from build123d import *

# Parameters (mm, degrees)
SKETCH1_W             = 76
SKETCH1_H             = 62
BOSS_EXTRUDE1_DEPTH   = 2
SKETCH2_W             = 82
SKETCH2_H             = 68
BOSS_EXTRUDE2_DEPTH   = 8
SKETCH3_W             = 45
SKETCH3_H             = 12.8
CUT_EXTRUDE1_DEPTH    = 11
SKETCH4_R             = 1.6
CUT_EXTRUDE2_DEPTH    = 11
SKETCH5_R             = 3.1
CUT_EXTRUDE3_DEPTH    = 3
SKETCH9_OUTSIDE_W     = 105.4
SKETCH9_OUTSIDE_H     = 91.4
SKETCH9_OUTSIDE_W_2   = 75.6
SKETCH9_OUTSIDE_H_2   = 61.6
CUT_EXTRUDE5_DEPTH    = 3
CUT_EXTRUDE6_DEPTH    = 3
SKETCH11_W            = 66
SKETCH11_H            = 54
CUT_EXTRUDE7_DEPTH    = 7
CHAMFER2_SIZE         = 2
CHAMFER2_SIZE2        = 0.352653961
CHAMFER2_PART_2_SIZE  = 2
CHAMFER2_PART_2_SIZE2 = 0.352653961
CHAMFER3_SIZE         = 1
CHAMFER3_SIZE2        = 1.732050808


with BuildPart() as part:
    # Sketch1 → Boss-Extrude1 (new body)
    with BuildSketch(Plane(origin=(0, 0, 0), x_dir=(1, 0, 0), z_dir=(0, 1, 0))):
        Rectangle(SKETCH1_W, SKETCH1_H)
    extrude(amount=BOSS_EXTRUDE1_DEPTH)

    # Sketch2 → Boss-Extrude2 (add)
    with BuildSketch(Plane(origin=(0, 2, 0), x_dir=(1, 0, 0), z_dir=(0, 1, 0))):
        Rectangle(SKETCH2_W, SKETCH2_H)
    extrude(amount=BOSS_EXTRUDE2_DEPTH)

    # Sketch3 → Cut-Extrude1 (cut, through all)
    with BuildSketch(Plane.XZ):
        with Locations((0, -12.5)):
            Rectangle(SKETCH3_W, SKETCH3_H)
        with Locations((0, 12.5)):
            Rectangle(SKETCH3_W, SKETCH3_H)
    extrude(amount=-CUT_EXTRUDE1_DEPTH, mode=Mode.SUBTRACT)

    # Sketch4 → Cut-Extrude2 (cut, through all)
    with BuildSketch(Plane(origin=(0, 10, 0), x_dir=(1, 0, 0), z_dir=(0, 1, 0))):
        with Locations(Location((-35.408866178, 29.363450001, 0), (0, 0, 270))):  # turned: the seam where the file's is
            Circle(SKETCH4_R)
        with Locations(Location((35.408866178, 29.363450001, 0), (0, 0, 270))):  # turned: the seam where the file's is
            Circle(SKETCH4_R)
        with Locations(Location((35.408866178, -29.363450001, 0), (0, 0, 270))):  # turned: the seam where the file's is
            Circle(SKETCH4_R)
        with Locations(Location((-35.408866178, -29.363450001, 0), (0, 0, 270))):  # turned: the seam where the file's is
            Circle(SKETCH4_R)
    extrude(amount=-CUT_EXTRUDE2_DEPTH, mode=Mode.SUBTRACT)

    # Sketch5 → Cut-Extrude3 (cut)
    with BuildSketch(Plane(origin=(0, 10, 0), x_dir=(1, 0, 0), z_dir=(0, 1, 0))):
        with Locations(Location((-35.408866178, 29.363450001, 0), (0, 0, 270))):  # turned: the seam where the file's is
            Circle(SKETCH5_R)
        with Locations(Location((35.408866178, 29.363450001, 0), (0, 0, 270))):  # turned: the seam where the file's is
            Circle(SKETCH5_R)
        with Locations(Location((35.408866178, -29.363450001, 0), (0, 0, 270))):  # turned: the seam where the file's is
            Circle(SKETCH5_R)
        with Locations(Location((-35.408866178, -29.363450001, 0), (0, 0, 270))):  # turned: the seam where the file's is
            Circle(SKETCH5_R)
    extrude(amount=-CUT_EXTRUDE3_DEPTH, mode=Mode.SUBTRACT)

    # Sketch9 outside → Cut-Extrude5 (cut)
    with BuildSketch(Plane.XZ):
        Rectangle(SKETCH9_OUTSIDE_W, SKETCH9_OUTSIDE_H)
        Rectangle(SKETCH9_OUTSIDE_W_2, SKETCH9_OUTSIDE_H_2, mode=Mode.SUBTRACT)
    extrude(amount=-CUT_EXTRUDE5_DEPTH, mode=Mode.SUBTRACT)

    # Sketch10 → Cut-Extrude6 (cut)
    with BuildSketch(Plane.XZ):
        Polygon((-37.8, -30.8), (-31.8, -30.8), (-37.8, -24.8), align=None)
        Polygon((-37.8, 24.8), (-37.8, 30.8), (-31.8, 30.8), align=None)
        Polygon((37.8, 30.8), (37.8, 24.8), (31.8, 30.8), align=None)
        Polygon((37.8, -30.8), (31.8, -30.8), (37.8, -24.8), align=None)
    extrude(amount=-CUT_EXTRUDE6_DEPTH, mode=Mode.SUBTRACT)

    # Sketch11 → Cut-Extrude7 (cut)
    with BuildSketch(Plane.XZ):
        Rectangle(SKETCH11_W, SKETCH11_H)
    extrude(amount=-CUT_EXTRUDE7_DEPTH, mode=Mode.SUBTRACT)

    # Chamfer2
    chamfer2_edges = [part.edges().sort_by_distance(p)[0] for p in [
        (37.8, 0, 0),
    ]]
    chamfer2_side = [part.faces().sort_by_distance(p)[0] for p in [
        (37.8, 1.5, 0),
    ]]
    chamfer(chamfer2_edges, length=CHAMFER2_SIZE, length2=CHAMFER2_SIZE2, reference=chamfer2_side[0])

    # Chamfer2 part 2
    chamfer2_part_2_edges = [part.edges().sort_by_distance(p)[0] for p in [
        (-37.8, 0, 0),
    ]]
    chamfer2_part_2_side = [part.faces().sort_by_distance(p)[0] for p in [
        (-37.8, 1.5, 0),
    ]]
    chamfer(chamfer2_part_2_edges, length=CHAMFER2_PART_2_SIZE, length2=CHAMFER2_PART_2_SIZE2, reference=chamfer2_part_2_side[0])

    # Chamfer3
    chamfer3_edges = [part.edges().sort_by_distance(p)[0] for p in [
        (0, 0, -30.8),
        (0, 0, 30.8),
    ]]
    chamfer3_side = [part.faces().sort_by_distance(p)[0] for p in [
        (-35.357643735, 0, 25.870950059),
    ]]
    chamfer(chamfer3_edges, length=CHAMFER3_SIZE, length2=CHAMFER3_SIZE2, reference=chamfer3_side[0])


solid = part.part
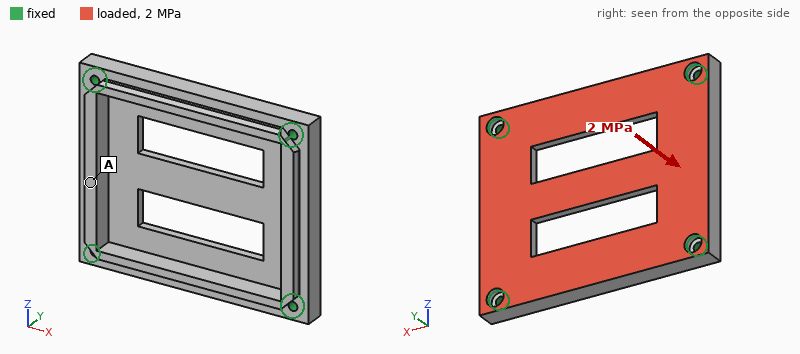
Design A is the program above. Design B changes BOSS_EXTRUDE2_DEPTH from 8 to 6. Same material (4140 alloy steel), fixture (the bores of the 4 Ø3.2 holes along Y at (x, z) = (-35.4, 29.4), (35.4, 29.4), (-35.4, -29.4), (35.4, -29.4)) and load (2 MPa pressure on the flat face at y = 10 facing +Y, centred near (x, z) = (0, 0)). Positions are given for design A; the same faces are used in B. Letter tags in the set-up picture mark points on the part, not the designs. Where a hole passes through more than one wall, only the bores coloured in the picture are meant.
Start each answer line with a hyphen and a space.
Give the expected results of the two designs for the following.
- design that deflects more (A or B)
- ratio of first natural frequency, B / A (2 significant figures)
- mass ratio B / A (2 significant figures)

- B
- 0.40
- 0.64
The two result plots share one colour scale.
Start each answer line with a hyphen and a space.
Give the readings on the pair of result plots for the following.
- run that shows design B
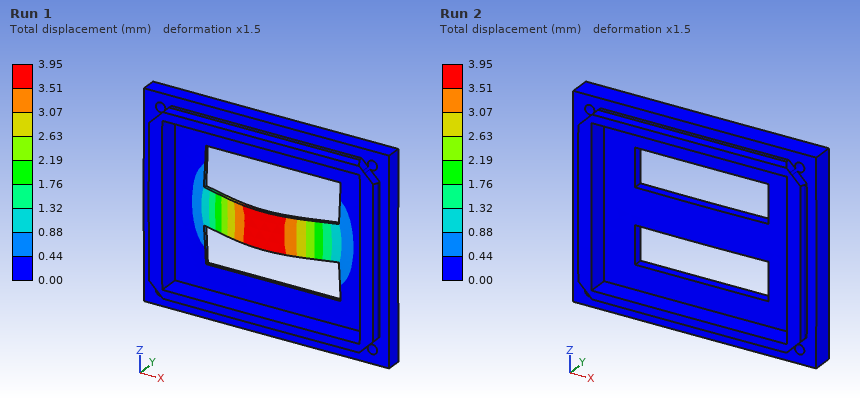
- Run 1
